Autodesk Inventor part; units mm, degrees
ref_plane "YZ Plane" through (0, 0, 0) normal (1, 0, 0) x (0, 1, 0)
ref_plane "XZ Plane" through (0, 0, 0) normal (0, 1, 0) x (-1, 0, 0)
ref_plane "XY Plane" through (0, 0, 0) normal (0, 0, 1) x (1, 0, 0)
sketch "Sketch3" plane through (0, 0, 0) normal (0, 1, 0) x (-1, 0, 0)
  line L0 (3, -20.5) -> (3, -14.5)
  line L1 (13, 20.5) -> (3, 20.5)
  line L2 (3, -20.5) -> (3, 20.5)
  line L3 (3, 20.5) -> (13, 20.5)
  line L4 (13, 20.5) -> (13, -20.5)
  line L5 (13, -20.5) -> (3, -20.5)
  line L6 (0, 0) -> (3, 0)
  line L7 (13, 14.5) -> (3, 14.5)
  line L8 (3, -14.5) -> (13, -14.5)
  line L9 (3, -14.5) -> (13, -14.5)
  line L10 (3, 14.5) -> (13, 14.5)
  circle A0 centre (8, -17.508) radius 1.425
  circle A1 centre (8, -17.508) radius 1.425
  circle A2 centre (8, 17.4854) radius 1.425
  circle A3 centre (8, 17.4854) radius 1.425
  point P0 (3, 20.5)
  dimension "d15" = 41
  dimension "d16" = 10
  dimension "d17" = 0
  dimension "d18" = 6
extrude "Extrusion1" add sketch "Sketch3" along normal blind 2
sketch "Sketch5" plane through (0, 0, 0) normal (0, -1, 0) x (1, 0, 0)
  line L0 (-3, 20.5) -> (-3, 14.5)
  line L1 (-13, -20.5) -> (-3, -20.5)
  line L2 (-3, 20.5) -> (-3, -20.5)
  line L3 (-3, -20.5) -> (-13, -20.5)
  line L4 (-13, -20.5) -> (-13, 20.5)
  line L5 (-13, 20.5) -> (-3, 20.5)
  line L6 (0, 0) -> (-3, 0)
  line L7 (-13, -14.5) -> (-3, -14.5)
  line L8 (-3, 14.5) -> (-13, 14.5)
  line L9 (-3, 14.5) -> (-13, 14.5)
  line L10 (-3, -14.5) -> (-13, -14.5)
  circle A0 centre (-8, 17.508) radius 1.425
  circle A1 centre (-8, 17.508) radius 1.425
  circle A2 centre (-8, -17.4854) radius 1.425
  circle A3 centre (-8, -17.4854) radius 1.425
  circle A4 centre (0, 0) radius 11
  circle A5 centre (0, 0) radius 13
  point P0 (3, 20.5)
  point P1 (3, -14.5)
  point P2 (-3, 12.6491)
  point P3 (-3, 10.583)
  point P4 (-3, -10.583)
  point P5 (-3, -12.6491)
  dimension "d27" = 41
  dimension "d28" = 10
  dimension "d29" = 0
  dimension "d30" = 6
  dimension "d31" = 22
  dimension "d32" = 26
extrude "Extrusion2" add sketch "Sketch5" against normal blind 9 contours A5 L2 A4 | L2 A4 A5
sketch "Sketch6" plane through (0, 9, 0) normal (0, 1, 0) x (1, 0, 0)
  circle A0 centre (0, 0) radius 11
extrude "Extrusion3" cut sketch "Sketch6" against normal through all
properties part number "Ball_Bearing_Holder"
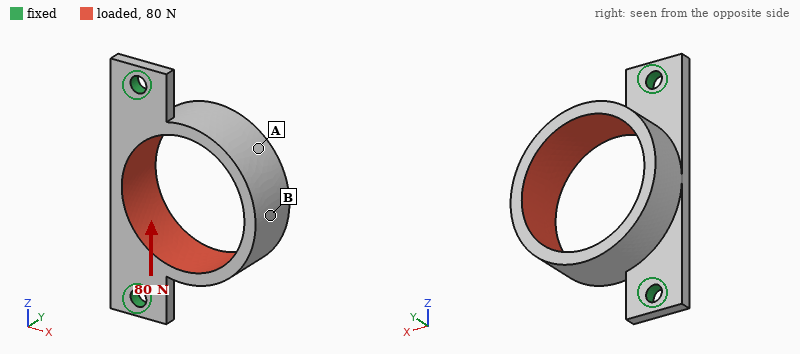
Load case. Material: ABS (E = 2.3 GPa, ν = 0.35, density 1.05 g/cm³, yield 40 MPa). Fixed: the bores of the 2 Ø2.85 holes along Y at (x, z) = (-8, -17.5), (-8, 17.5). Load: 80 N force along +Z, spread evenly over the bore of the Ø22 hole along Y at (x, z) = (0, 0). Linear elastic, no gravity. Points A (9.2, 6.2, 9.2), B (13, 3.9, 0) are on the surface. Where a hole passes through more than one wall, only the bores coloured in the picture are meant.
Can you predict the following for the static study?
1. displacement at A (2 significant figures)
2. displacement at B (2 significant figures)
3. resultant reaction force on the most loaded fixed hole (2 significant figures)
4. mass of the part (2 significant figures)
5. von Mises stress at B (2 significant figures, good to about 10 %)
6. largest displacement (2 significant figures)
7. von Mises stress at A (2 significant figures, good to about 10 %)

0.39 mm
0.37 mm
44 N
1.9 g
2.7 MPa
0.43 mm
8.6 MPa
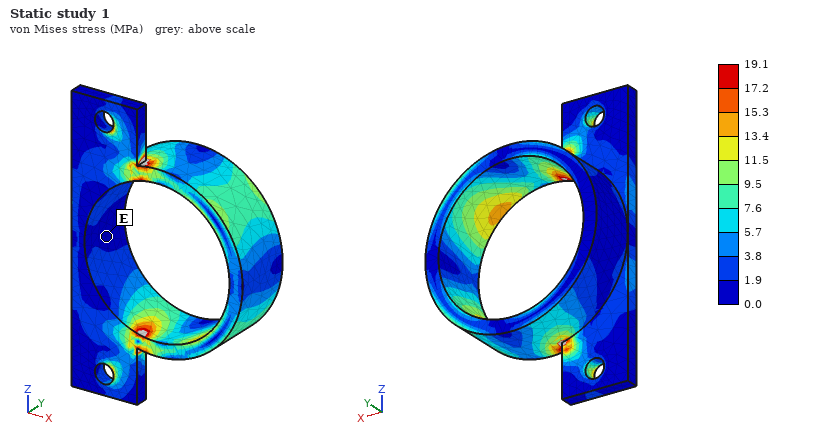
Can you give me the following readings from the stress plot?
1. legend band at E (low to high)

0.0 to 1.9 MPa
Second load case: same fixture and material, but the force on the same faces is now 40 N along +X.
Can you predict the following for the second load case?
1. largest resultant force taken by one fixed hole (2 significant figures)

21 N
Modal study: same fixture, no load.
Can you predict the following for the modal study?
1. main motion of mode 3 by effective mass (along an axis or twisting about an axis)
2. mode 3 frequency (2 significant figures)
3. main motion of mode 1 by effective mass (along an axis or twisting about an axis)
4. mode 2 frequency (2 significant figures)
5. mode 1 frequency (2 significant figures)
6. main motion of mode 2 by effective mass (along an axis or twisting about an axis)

twisting about X
3000 Hz
along Y
2000 Hz
870 Hz
along Z
